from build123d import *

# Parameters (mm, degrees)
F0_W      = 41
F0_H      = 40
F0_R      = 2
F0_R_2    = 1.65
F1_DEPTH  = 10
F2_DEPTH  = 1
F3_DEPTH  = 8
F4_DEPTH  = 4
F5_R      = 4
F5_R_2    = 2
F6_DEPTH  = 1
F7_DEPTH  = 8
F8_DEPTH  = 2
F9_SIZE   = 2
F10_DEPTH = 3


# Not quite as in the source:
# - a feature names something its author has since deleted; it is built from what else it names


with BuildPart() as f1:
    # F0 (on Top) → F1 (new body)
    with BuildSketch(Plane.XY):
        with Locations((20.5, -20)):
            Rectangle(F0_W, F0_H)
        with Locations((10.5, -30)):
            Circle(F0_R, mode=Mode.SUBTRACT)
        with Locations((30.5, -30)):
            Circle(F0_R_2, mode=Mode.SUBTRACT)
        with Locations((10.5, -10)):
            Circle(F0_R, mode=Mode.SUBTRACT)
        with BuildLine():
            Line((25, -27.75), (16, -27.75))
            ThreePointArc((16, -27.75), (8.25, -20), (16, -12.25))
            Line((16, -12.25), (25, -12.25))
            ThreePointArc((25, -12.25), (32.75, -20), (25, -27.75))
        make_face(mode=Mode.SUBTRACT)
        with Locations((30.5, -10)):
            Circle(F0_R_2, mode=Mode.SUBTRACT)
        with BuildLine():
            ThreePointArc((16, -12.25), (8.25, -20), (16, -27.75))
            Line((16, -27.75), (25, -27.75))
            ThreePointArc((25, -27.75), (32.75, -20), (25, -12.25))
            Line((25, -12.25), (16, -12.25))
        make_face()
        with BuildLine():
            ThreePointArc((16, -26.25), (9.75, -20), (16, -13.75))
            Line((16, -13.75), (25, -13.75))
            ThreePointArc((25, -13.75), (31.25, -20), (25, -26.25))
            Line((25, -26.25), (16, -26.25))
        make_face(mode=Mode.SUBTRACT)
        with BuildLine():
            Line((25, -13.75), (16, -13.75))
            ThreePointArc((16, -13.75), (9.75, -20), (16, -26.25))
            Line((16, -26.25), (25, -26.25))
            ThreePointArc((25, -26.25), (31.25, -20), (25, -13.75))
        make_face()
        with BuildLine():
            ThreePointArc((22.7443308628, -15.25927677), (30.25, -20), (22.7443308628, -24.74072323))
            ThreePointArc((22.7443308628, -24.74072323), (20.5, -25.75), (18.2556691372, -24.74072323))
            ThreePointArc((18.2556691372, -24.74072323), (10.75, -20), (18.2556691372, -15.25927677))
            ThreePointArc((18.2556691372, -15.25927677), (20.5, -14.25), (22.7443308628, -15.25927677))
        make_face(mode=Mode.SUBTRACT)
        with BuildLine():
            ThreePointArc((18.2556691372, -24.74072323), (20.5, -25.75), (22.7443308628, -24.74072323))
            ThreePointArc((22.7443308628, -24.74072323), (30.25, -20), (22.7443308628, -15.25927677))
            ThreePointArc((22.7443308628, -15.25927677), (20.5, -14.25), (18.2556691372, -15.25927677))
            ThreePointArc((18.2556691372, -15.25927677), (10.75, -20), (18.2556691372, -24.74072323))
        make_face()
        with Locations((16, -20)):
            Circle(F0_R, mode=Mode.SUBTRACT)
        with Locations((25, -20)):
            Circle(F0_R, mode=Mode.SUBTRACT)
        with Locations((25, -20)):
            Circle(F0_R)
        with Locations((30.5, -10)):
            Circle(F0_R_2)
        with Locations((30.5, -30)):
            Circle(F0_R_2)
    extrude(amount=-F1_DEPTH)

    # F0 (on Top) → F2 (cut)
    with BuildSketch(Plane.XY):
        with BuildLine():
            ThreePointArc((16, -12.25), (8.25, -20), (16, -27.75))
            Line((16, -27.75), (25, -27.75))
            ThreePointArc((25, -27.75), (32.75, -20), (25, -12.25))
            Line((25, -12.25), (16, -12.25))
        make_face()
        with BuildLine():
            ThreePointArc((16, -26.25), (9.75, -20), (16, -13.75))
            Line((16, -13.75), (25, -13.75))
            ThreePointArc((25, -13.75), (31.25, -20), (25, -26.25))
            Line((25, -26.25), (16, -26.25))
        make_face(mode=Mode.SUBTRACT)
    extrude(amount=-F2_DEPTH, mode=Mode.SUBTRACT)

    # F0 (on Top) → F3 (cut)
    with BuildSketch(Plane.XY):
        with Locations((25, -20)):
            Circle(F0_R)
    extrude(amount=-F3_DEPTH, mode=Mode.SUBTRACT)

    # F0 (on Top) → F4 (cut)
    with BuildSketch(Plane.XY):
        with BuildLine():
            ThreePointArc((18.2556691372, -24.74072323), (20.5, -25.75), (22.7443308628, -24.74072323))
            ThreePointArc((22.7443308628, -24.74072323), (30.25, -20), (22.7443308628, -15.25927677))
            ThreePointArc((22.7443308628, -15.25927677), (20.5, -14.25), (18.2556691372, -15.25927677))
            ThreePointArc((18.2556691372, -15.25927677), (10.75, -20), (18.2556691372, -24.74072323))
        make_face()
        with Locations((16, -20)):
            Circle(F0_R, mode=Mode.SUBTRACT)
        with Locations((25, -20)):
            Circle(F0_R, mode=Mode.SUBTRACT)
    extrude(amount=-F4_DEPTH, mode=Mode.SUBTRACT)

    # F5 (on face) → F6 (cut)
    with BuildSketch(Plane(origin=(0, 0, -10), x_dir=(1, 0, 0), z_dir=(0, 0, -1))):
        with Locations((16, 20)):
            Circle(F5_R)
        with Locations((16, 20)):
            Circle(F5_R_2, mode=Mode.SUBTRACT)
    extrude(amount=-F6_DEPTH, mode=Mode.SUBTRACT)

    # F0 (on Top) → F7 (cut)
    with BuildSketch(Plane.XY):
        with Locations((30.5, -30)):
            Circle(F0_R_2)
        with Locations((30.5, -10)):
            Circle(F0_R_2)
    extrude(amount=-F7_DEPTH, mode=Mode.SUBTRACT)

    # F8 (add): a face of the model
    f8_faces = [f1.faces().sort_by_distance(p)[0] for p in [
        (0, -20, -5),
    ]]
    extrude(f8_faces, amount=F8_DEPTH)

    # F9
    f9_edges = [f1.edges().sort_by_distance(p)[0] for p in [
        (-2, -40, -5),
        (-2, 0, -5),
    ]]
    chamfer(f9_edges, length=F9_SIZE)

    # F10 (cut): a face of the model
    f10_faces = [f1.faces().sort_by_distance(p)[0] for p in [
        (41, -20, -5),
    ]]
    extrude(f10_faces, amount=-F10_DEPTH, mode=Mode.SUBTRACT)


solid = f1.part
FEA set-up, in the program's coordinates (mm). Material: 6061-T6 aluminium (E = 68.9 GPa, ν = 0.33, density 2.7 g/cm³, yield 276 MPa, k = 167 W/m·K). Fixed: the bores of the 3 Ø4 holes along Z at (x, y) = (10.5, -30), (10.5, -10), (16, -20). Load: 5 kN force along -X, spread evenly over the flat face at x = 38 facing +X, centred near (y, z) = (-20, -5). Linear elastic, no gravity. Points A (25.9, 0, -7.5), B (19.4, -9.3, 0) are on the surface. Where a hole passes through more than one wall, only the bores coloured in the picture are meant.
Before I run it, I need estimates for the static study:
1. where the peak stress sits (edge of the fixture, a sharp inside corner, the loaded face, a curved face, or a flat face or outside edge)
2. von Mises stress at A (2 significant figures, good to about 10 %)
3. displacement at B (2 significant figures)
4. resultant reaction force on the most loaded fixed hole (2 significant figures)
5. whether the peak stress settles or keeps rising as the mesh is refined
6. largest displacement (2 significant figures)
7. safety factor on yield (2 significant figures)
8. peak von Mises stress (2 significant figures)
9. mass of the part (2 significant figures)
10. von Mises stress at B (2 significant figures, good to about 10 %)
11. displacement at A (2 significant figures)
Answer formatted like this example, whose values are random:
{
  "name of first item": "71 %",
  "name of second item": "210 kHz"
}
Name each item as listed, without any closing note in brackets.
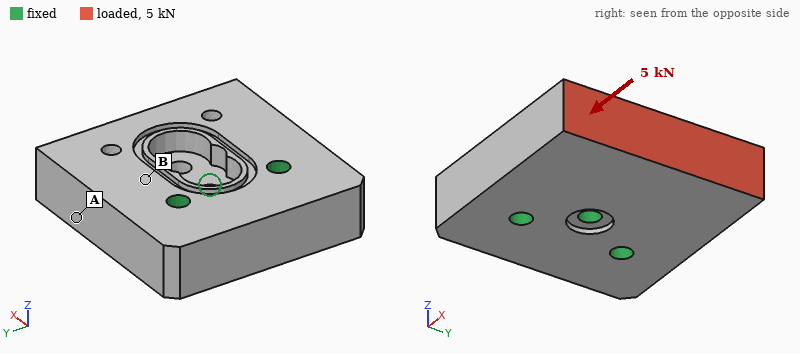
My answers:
{
  "where the peak stress sits": "a curved face",
  "von Mises stress at A": "7.4 MPa",
  "displacement at B": "2.8 µm",
  "resultant reaction force on the most loaded fixed hole": "2.0 kN",
  "whether the peak stress settles or keeps rising as the mesh is refined": "settles",
  "largest displacement": "10 µm",
  "safety factor on yield": "4.4",
  "peak von Mises stress": "62 MPa",
  "mass of the part": "39 g",
  "von Mises stress at B": "20 MPa",
  "displacement at A": "3.9 µm"
}
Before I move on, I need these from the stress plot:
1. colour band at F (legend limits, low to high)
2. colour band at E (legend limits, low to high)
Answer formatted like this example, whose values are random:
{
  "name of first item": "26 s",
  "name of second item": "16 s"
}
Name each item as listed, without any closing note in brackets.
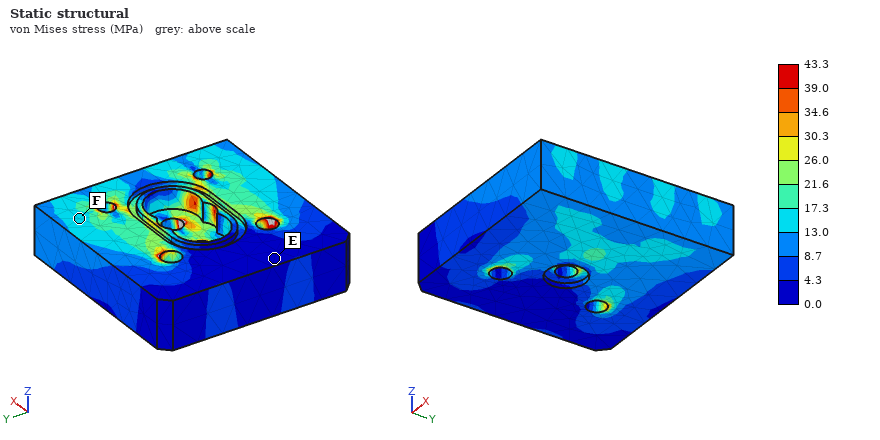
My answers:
{
  "colour band at F": "13.0 to 17.3 MPa",
  "colour band at E": "0.0 to 4.3 MPa"
}
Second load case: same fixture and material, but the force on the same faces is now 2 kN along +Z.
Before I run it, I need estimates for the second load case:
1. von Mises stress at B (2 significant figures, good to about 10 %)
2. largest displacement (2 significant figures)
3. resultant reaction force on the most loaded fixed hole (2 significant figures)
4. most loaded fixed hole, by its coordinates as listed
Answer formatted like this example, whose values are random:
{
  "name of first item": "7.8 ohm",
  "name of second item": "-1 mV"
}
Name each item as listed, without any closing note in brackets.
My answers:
{
  "von Mises stress at B": "74 MPa",
  "largest displacement": "78 µm",
  "resultant reaction force on the most loaded fixed hole": "1.9 kN",
  "most loaded fixed hole, by its coordinates as listed": "(16, -20)"
}
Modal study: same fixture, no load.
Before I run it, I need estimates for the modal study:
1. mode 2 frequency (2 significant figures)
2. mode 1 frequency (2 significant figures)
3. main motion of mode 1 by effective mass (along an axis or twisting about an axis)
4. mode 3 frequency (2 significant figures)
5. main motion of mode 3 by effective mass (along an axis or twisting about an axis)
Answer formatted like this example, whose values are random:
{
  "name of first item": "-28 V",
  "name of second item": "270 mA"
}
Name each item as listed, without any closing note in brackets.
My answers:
{
  "mode 2 frequency": "14 kHz",
  "mode 1 frequency": "9700 Hz",
  "main motion of mode 1 by effective mass": "along Z",
  "mode 3 frequency": "19 kHz",
  "main motion of mode 3 by effective mass": "along Y"
}
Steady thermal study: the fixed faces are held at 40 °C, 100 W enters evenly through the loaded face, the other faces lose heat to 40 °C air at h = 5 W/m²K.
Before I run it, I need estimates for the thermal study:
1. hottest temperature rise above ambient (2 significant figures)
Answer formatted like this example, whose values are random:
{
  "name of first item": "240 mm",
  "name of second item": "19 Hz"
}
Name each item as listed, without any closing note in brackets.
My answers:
{
  "hottest temperature rise above ambient": "45 K"
}
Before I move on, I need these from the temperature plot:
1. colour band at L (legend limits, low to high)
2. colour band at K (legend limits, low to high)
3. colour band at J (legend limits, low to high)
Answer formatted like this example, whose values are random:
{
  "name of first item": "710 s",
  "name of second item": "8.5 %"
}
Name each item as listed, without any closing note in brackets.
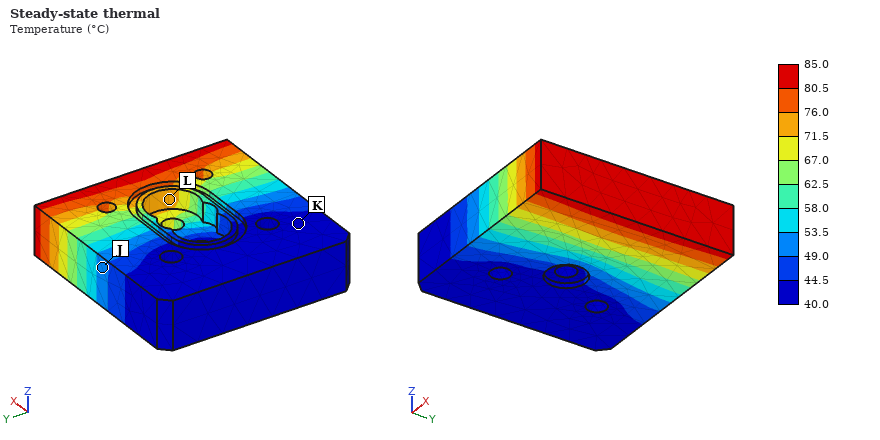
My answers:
{
  "colour band at L": "71.5 to 76.0 °C",
  "colour band at K": "40.0 to 44.5 °C",
  "colour band at J": "49.0 to 53.5 °C"
}
